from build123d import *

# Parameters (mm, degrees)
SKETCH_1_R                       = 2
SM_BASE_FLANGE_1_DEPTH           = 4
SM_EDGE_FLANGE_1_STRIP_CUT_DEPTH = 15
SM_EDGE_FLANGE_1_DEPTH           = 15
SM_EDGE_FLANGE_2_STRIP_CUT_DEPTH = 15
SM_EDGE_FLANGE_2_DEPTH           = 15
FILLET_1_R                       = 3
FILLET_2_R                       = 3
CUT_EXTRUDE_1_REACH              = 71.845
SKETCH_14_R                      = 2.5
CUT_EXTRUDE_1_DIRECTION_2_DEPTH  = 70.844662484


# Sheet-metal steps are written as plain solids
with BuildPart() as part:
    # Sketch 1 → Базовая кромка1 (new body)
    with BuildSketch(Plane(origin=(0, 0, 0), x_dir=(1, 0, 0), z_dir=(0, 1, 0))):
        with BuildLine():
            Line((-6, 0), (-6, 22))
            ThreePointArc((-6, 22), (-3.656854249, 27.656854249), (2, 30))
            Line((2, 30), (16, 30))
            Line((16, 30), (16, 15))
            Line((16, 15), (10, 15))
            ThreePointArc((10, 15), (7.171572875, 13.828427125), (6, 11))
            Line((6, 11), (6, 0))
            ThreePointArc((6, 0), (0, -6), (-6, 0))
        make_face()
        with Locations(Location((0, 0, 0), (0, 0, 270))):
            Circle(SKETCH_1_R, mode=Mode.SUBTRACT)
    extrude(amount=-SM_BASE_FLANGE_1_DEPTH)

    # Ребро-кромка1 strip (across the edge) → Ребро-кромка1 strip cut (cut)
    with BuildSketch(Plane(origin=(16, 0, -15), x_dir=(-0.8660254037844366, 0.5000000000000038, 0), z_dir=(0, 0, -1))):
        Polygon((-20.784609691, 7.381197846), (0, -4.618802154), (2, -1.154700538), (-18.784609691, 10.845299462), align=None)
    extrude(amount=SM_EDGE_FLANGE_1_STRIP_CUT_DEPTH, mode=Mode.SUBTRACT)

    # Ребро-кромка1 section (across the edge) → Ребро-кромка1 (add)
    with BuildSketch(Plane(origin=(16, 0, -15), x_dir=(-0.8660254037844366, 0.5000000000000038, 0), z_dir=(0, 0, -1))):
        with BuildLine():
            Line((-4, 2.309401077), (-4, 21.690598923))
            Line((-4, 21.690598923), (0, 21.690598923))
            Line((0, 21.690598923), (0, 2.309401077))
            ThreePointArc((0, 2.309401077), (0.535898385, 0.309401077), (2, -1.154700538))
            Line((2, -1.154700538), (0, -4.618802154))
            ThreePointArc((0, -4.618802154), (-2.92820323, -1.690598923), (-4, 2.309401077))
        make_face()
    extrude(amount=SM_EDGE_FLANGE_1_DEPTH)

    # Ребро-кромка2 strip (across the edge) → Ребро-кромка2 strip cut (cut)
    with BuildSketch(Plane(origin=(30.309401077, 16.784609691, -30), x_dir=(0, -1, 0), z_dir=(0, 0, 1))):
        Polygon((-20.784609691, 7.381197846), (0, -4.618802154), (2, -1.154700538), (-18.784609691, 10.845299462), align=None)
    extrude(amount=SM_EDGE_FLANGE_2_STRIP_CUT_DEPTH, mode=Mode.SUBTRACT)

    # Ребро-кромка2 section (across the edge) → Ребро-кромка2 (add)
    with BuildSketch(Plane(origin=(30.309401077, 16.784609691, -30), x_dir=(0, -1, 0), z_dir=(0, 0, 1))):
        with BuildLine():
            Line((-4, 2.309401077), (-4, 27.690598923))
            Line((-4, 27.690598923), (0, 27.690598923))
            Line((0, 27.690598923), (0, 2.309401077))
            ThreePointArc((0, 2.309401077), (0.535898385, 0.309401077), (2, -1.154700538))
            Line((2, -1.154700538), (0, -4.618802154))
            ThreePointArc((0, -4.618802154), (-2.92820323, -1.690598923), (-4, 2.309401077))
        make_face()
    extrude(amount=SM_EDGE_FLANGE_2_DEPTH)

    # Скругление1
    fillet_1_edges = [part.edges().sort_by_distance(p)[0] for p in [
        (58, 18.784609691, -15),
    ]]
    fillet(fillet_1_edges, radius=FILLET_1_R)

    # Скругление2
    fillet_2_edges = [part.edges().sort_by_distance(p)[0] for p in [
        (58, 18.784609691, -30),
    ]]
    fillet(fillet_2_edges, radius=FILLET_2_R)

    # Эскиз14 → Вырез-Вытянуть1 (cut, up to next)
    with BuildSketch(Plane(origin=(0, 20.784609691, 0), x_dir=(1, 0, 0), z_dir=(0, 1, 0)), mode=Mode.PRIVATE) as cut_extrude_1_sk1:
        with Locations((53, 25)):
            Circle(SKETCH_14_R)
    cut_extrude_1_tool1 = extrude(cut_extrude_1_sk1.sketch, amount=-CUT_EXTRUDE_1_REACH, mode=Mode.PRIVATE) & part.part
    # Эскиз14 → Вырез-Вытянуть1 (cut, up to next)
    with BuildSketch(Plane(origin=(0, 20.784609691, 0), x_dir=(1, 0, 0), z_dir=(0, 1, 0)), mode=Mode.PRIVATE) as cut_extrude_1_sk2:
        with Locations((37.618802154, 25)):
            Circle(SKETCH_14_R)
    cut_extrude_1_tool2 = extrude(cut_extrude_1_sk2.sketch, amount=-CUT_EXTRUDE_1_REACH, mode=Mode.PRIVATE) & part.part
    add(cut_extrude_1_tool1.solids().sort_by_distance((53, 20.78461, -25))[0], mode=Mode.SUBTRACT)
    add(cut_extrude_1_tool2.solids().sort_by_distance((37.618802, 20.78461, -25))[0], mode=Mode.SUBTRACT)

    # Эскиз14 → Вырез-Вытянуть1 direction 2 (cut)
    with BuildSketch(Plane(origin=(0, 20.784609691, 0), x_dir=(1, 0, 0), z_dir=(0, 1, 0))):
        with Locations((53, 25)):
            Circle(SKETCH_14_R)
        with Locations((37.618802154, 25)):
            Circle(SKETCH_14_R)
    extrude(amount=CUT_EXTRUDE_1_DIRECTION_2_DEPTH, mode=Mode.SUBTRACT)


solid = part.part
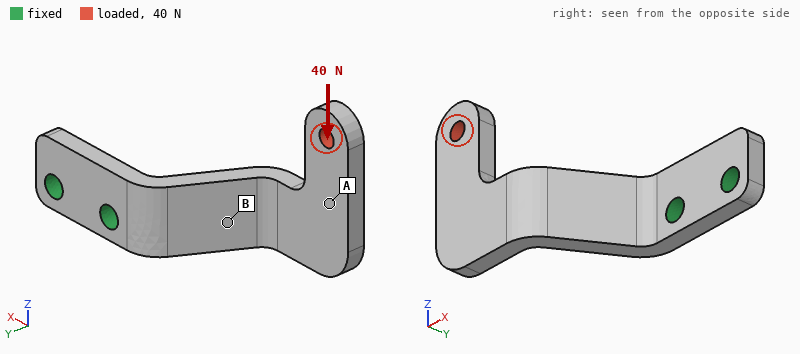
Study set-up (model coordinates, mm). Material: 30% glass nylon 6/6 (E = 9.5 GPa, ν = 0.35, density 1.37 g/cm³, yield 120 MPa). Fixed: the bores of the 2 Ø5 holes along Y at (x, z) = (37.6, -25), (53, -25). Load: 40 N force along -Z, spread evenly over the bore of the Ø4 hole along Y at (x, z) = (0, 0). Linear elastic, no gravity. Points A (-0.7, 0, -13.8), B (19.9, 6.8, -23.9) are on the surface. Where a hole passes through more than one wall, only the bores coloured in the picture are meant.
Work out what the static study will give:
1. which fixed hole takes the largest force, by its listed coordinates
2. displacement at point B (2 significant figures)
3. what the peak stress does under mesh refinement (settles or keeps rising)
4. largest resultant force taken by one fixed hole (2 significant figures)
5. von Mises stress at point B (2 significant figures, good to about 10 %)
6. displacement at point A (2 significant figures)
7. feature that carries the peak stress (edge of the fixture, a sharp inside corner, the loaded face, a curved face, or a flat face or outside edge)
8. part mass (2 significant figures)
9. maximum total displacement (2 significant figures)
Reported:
(37.6, -25)
0.092 mm
keeps rising
97 N
16 MPa
0.36 mm
edge of the fixture
7.1 g
0.51 mm
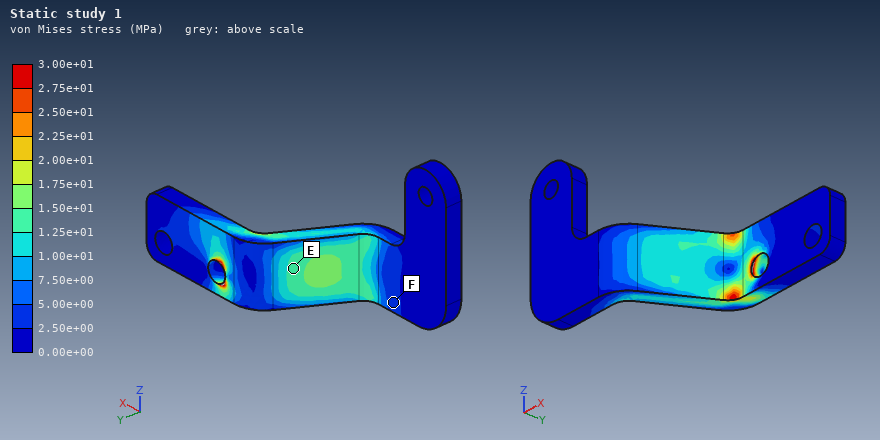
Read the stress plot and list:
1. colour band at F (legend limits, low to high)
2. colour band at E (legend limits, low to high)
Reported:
2.50e+00 to 5.00e+00 MPa
1.25e+01 to 1.50e+01 MPa
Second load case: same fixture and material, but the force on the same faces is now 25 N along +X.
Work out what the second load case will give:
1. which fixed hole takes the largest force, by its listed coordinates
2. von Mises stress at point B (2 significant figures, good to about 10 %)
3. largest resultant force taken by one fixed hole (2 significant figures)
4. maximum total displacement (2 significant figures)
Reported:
(53, -25)
13 MPa
29 N
0.83 mm
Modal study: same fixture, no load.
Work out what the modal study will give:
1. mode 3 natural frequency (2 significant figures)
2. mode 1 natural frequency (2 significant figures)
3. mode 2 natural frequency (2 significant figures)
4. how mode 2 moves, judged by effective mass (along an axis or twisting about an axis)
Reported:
1500 Hz
480 Hz
980 Hz
along Z
